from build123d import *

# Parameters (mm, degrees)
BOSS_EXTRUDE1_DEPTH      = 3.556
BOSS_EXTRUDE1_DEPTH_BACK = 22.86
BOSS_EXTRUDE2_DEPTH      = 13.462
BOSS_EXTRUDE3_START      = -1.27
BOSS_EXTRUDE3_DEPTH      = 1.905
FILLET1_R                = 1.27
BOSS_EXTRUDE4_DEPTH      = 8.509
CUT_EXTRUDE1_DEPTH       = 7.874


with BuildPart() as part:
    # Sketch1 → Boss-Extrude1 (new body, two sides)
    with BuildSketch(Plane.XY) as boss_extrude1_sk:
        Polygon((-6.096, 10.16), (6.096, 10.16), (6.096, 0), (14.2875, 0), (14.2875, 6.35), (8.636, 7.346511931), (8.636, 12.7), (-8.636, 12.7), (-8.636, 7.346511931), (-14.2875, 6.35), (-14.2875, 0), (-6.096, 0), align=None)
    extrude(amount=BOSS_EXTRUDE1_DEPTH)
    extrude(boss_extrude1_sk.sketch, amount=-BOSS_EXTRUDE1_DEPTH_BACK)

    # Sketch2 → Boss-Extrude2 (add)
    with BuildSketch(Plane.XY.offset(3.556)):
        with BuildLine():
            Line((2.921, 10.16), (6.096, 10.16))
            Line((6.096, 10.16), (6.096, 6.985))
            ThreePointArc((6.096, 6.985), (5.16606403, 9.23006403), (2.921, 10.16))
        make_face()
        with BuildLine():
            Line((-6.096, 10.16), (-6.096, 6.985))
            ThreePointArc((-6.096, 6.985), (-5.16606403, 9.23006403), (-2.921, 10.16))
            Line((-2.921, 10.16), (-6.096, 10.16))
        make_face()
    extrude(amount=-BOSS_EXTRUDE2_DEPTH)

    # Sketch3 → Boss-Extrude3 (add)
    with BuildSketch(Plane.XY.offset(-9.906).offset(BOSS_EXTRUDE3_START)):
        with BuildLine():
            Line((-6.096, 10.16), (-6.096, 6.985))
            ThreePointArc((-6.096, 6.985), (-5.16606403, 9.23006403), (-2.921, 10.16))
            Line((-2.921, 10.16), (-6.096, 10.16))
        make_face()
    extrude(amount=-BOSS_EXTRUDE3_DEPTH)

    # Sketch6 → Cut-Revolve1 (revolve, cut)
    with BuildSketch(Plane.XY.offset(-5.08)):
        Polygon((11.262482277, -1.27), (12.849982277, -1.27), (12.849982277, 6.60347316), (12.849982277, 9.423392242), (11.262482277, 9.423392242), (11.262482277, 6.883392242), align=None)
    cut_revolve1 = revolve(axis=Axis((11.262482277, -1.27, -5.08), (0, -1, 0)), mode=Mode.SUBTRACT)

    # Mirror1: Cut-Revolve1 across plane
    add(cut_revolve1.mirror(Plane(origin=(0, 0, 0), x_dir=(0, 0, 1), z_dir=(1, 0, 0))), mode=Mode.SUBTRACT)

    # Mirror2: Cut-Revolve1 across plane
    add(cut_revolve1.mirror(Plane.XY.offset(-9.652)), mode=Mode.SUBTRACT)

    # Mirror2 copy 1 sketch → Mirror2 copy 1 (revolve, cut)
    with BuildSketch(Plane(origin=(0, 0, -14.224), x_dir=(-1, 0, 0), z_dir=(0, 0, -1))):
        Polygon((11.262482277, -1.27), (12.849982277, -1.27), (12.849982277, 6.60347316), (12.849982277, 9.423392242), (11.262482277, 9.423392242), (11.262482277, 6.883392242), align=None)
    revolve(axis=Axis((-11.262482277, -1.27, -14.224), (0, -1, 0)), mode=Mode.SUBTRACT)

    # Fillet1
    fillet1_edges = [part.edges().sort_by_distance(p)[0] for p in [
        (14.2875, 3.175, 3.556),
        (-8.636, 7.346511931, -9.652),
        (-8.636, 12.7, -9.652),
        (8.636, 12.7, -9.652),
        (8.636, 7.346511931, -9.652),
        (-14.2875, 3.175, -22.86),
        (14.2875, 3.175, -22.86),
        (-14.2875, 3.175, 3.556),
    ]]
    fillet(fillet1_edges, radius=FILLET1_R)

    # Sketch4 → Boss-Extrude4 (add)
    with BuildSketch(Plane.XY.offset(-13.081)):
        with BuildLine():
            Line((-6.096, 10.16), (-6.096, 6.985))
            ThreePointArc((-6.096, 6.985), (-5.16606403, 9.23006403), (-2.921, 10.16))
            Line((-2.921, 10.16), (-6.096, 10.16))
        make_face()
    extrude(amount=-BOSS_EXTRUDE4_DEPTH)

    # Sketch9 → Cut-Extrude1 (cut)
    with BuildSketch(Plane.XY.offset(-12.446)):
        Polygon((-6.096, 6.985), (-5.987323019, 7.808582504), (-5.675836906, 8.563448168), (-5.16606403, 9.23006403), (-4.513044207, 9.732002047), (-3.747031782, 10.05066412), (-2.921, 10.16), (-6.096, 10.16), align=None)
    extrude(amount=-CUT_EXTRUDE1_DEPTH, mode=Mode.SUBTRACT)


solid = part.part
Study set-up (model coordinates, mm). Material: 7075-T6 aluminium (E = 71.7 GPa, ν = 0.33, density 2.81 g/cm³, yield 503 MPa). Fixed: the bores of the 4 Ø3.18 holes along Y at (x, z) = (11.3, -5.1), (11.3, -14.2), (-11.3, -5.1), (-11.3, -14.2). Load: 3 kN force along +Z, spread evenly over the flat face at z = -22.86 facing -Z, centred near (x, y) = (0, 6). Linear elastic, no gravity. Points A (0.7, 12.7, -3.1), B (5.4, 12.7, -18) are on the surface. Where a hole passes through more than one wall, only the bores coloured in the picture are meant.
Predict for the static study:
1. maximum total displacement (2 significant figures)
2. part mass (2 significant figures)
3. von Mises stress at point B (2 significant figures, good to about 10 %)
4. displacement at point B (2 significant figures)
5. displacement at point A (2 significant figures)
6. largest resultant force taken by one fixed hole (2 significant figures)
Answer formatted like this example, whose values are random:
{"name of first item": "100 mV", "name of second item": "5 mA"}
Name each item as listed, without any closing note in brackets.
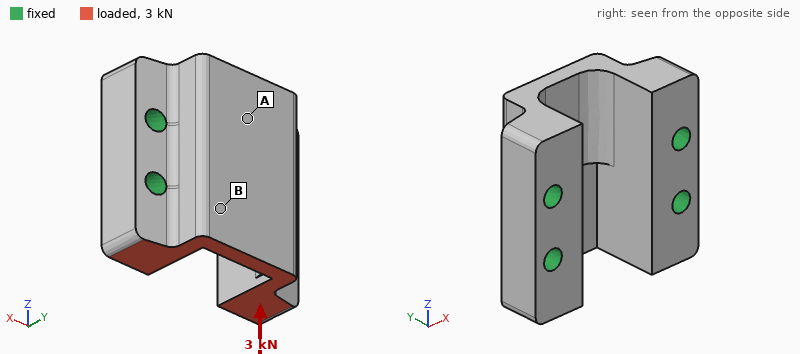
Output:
{"maximum total displacement": "9.2 µm", "part mass": "12 g", "von Mises stress at point B": "21 MPa", "displacement at point B": "6.4 µm", "displacement at point A": "4.0 µm", "largest resultant force taken by one fixed hole": "1.1 kN"}
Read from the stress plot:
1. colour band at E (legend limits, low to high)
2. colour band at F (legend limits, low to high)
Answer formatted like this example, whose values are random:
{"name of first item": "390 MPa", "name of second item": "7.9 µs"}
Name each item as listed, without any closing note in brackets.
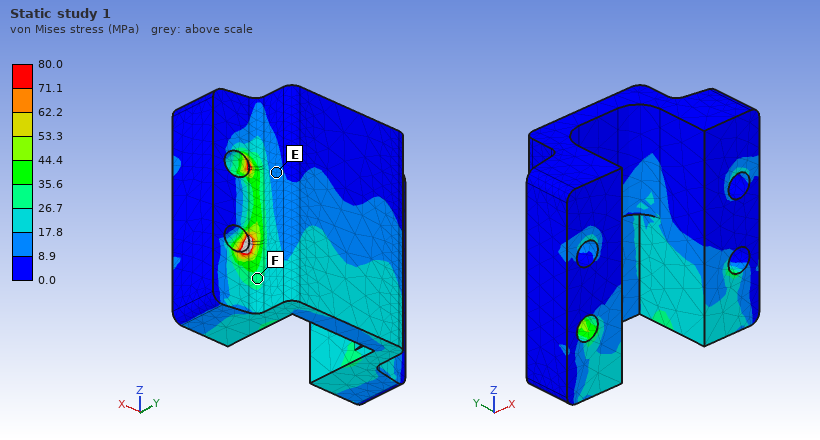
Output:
{"colour band at E": "8.9 to 17.8 MPa", "colour band at F": "26.7 to 35.6 MPa"}
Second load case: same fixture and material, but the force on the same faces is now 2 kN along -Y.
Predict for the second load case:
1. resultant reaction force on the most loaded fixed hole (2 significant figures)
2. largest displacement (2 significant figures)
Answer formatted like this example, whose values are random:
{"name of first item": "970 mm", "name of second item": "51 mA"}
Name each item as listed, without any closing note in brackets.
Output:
{"resultant reaction force on the most loaded fixed hole": "1.3 kN", "largest displacement": "30 µm"}
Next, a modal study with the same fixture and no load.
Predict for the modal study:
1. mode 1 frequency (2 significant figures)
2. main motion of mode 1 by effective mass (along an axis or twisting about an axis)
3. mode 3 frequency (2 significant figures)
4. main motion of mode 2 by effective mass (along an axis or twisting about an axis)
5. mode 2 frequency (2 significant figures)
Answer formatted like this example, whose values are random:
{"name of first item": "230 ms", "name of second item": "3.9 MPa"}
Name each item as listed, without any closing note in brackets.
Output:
{"mode 1 frequency": "35 kHz", "main motion of mode 1 by effective mass": "along Z", "mode 3 frequency": "41 kHz", "main motion of mode 2 by effective mass": "along X", "mode 2 frequency": "37 kHz"}
